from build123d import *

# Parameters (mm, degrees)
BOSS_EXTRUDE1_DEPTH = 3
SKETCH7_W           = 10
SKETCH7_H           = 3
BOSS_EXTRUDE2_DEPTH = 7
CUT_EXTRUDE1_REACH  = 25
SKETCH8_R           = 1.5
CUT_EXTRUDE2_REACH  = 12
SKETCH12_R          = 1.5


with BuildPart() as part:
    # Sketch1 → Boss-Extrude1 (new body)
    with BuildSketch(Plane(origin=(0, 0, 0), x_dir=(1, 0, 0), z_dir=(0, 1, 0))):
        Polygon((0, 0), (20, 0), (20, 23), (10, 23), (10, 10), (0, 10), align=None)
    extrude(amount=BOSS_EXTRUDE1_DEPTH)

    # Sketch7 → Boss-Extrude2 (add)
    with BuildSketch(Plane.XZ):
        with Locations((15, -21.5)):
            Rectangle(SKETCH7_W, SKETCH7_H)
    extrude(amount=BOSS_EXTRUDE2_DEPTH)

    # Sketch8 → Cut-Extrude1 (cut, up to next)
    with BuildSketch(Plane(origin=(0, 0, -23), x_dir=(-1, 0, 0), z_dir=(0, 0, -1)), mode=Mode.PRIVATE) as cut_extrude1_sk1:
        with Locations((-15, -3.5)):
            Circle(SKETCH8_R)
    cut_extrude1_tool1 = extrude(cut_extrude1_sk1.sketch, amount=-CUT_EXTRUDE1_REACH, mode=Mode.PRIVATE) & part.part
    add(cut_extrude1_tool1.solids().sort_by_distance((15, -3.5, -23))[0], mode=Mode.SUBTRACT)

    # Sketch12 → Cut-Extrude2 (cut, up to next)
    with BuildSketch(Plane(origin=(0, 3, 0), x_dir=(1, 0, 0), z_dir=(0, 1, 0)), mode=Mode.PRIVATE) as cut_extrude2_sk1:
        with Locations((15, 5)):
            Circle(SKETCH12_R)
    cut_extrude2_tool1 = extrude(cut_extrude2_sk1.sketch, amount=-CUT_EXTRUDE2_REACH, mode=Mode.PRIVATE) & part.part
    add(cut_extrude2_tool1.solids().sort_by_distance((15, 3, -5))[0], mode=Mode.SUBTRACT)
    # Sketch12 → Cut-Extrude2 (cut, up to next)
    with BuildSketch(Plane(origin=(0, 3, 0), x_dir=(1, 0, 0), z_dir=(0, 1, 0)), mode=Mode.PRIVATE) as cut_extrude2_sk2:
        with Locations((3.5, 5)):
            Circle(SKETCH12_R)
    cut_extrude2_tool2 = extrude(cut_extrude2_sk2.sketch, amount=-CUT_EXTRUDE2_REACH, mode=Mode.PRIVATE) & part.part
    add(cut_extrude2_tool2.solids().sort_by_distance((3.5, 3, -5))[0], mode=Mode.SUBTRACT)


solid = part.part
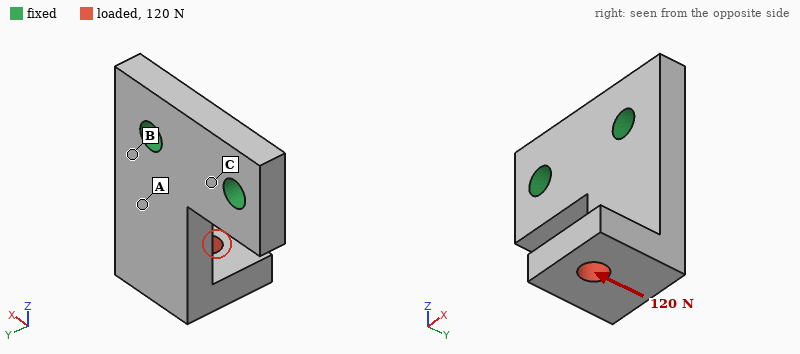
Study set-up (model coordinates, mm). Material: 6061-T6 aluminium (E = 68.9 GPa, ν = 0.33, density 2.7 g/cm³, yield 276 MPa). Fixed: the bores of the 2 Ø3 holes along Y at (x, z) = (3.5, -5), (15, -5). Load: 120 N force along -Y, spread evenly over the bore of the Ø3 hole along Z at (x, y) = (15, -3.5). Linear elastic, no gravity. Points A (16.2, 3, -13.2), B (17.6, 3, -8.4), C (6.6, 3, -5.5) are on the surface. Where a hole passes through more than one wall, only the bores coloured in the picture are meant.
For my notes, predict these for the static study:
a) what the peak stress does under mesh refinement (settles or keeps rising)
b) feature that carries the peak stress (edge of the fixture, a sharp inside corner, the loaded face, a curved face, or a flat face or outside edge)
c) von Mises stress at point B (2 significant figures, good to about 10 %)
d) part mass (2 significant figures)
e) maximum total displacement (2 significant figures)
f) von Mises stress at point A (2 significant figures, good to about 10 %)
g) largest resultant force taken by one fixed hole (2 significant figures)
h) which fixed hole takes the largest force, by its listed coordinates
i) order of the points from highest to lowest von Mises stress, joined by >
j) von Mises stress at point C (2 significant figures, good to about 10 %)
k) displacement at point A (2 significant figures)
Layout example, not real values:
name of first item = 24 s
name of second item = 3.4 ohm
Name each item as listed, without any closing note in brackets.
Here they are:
what the peak stress does under mesh refinement = keeps rising
feature that carries the peak stress = edge of the fixture
von Mises stress at point B = 85 MPa
part mass = 3.1 g
maximum total displacement = 0.14 mm
von Mises stress at point A = 62 MPa
largest resultant force taken by one fixed hole = 130 N
which fixed hole takes the largest force, by its listed coordinates = (15, -5)
order of the points from highest to lowest von Mises stress, joined by > = B > A > C
von Mises stress at point C = 20 MPa
displacement at point A = 0.030 mm
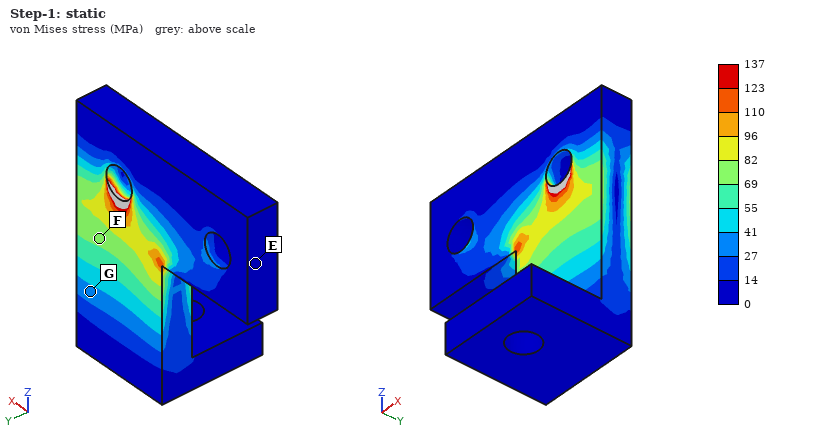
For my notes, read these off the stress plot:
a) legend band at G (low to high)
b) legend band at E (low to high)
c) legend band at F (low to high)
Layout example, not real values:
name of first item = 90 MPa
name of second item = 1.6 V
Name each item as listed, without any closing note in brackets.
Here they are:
legend band at G = 27 to 41 MPa
legend band at E = 0 to 14 MPa
legend band at F = 69 to 82 MPa
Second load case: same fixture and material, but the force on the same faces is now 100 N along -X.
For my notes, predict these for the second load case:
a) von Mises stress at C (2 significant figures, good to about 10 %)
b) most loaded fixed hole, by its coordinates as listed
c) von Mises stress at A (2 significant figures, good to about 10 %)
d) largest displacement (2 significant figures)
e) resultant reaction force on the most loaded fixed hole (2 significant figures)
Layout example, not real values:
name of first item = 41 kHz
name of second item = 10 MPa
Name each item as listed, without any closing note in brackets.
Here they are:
von Mises stress at C = 15 MPa
most loaded fixed hole, by its coordinates as listed = (3.5, -5)
von Mises stress at A = 24 MPa
largest displacement = 44 µm
resultant reaction force on the most loaded fixed hole = 130 N
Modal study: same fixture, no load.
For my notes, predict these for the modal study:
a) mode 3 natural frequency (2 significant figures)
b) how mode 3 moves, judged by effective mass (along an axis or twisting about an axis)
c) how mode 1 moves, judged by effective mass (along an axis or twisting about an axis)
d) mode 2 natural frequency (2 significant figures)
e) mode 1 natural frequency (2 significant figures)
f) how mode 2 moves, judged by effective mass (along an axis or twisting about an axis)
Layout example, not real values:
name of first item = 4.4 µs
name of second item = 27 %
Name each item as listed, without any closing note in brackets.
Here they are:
mode 3 natural frequency = 19 kHz
how mode 3 moves, judged by effective mass = along X
how mode 1 moves, judged by effective mass = along Y
mode 2 natural frequency = 11 kHz
mode 1 natural frequency = 5300 Hz
how mode 2 moves, judged by effective mass = along X
